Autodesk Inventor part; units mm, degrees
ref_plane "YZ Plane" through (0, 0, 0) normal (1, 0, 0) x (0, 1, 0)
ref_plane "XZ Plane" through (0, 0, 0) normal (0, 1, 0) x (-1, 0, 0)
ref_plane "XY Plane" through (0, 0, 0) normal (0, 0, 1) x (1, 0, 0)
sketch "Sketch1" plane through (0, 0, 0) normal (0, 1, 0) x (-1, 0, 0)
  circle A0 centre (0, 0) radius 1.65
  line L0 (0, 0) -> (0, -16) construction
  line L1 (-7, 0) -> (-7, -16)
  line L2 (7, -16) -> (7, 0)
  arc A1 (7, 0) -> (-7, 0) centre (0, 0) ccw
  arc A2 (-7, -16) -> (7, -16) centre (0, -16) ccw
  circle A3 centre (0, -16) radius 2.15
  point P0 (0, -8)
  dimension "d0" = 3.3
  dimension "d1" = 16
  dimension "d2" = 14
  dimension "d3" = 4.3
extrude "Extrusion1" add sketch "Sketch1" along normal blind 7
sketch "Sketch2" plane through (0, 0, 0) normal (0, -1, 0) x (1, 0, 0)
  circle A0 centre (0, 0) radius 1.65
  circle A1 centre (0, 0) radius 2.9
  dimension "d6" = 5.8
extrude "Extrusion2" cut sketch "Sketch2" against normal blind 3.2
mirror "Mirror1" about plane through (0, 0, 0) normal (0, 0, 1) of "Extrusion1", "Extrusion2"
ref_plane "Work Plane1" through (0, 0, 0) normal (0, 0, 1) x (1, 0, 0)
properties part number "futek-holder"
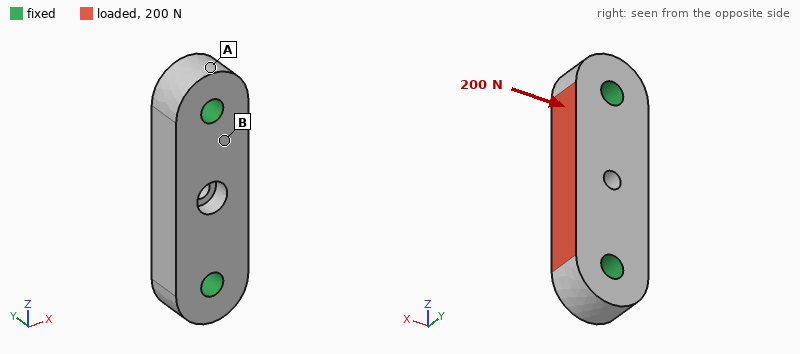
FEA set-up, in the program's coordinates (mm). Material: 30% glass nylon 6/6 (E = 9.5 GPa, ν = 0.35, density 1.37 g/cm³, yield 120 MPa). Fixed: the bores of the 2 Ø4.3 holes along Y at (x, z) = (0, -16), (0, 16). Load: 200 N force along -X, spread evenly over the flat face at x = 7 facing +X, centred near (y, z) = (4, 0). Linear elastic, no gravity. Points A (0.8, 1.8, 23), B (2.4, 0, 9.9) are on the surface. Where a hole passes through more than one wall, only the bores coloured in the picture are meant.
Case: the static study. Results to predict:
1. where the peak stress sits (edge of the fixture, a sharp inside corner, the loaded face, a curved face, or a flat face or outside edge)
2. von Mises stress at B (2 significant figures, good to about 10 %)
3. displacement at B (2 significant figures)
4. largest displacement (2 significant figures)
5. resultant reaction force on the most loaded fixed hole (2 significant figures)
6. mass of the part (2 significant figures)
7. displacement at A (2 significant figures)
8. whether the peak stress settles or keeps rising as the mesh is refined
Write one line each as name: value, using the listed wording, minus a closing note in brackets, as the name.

where the peak stress sits: edge of the fixture
von Mises stress at B: 1.6 MPa
displacement at B: 2.5 µm
largest displacement: 5.2 µm
resultant reaction force on the most loaded fixed hole: 100 N
mass of the part: 5.3 g
displacement at A: 0.85 µm
whether the peak stress settles or keeps rising as the mesh is refined: keeps rising
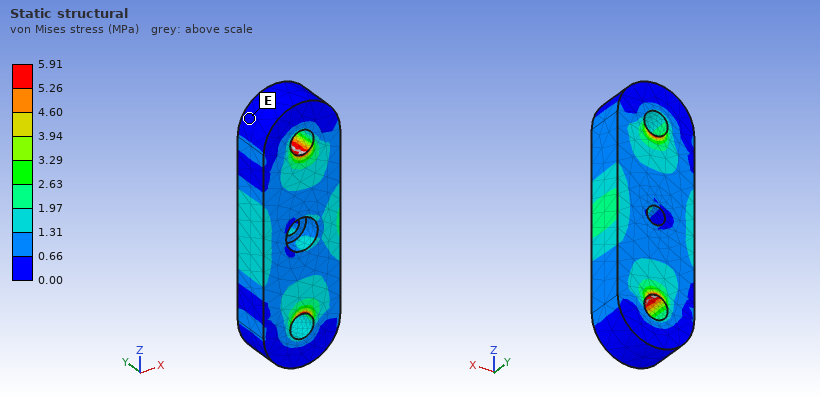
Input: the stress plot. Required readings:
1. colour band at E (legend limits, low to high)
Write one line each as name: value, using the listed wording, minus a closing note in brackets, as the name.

colour band at E: 0.00 to 0.66 MPa
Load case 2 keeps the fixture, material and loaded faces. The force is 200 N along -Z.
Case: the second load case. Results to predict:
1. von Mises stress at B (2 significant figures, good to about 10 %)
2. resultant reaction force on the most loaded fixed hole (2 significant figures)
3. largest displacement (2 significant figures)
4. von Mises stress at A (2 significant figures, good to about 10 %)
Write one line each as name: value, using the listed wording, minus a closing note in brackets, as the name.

von Mises stress at B: 1.5 MPa
resultant reaction force on the most loaded fixed hole: 110 N
largest displacement: 2.2 µm
von Mises stress at A: 0.44 MPa
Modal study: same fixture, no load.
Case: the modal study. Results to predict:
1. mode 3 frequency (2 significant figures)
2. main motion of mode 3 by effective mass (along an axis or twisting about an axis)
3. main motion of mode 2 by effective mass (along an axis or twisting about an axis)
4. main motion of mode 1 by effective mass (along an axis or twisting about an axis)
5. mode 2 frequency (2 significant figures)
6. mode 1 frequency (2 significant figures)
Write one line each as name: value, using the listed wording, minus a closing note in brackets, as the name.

mode 3 frequency: 20 kHz
main motion of mode 3 by effective mass: twisting about Z
main motion of mode 2 by effective mass: along X
main motion of mode 1 by effective mass: along Y
mode 2 frequency: 18 kHz
mode 1 frequency: 15 kHz
